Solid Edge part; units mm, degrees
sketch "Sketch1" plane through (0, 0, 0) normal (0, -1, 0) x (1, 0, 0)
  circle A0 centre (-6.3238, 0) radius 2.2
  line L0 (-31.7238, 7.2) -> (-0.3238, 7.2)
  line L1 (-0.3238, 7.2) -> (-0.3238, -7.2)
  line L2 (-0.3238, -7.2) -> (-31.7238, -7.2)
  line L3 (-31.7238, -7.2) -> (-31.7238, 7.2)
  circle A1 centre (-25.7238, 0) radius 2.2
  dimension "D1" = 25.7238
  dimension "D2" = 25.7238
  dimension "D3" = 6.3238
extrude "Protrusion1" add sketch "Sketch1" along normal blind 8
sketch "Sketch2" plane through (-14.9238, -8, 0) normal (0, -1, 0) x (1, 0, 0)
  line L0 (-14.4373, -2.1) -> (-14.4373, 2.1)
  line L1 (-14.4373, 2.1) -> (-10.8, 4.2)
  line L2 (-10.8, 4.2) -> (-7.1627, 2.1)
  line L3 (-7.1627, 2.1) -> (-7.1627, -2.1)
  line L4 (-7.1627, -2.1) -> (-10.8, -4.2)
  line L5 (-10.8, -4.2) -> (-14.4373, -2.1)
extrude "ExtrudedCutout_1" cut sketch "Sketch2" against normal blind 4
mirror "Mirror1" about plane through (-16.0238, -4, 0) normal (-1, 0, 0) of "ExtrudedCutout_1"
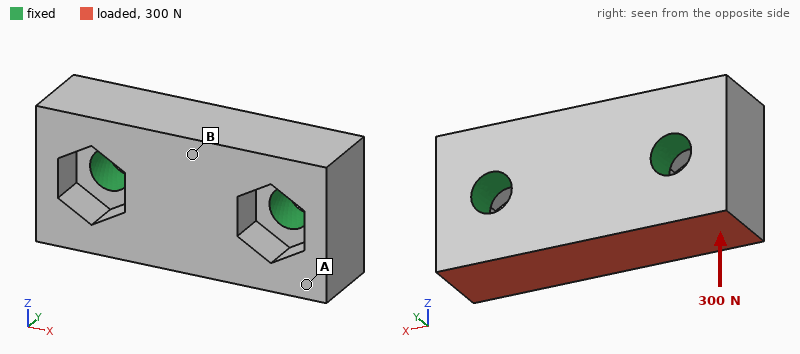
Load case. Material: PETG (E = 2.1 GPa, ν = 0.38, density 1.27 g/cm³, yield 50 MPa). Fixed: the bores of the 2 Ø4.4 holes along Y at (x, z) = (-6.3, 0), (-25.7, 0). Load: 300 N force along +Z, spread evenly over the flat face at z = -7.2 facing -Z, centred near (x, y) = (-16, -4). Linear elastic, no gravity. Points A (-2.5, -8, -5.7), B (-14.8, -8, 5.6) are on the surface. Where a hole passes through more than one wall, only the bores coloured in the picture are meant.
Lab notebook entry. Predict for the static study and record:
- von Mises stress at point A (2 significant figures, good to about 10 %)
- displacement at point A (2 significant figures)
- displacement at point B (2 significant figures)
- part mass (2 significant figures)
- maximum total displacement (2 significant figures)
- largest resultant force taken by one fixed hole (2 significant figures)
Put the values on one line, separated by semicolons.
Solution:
1.7 MPa; 27 µm; 26 µm; 4.0 g; 35 µm; 150 N
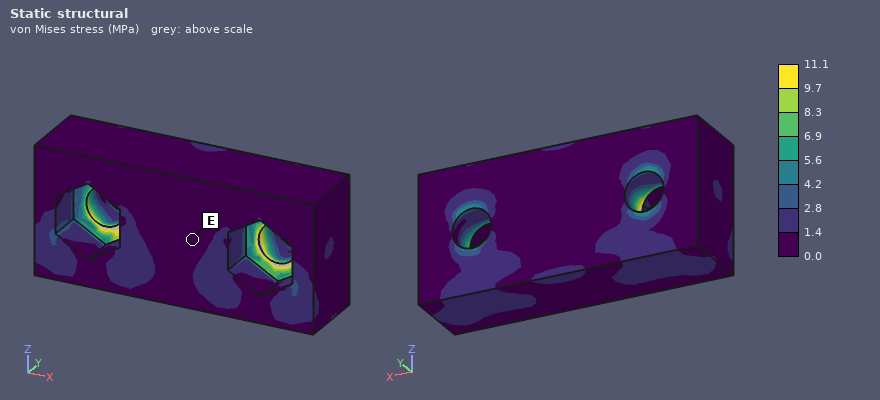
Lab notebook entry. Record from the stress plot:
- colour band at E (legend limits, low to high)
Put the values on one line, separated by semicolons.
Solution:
0.0 to 1.4 MPa
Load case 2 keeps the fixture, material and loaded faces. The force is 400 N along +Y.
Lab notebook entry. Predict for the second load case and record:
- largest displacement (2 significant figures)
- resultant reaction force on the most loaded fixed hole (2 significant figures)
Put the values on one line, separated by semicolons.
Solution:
0.14 mm; 200 N
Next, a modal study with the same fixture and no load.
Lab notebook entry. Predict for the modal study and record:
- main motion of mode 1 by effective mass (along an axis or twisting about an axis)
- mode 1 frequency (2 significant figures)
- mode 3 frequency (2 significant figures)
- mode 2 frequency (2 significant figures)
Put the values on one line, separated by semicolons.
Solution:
along Z; 7900 Hz; 12 kHz; 12 kHz
